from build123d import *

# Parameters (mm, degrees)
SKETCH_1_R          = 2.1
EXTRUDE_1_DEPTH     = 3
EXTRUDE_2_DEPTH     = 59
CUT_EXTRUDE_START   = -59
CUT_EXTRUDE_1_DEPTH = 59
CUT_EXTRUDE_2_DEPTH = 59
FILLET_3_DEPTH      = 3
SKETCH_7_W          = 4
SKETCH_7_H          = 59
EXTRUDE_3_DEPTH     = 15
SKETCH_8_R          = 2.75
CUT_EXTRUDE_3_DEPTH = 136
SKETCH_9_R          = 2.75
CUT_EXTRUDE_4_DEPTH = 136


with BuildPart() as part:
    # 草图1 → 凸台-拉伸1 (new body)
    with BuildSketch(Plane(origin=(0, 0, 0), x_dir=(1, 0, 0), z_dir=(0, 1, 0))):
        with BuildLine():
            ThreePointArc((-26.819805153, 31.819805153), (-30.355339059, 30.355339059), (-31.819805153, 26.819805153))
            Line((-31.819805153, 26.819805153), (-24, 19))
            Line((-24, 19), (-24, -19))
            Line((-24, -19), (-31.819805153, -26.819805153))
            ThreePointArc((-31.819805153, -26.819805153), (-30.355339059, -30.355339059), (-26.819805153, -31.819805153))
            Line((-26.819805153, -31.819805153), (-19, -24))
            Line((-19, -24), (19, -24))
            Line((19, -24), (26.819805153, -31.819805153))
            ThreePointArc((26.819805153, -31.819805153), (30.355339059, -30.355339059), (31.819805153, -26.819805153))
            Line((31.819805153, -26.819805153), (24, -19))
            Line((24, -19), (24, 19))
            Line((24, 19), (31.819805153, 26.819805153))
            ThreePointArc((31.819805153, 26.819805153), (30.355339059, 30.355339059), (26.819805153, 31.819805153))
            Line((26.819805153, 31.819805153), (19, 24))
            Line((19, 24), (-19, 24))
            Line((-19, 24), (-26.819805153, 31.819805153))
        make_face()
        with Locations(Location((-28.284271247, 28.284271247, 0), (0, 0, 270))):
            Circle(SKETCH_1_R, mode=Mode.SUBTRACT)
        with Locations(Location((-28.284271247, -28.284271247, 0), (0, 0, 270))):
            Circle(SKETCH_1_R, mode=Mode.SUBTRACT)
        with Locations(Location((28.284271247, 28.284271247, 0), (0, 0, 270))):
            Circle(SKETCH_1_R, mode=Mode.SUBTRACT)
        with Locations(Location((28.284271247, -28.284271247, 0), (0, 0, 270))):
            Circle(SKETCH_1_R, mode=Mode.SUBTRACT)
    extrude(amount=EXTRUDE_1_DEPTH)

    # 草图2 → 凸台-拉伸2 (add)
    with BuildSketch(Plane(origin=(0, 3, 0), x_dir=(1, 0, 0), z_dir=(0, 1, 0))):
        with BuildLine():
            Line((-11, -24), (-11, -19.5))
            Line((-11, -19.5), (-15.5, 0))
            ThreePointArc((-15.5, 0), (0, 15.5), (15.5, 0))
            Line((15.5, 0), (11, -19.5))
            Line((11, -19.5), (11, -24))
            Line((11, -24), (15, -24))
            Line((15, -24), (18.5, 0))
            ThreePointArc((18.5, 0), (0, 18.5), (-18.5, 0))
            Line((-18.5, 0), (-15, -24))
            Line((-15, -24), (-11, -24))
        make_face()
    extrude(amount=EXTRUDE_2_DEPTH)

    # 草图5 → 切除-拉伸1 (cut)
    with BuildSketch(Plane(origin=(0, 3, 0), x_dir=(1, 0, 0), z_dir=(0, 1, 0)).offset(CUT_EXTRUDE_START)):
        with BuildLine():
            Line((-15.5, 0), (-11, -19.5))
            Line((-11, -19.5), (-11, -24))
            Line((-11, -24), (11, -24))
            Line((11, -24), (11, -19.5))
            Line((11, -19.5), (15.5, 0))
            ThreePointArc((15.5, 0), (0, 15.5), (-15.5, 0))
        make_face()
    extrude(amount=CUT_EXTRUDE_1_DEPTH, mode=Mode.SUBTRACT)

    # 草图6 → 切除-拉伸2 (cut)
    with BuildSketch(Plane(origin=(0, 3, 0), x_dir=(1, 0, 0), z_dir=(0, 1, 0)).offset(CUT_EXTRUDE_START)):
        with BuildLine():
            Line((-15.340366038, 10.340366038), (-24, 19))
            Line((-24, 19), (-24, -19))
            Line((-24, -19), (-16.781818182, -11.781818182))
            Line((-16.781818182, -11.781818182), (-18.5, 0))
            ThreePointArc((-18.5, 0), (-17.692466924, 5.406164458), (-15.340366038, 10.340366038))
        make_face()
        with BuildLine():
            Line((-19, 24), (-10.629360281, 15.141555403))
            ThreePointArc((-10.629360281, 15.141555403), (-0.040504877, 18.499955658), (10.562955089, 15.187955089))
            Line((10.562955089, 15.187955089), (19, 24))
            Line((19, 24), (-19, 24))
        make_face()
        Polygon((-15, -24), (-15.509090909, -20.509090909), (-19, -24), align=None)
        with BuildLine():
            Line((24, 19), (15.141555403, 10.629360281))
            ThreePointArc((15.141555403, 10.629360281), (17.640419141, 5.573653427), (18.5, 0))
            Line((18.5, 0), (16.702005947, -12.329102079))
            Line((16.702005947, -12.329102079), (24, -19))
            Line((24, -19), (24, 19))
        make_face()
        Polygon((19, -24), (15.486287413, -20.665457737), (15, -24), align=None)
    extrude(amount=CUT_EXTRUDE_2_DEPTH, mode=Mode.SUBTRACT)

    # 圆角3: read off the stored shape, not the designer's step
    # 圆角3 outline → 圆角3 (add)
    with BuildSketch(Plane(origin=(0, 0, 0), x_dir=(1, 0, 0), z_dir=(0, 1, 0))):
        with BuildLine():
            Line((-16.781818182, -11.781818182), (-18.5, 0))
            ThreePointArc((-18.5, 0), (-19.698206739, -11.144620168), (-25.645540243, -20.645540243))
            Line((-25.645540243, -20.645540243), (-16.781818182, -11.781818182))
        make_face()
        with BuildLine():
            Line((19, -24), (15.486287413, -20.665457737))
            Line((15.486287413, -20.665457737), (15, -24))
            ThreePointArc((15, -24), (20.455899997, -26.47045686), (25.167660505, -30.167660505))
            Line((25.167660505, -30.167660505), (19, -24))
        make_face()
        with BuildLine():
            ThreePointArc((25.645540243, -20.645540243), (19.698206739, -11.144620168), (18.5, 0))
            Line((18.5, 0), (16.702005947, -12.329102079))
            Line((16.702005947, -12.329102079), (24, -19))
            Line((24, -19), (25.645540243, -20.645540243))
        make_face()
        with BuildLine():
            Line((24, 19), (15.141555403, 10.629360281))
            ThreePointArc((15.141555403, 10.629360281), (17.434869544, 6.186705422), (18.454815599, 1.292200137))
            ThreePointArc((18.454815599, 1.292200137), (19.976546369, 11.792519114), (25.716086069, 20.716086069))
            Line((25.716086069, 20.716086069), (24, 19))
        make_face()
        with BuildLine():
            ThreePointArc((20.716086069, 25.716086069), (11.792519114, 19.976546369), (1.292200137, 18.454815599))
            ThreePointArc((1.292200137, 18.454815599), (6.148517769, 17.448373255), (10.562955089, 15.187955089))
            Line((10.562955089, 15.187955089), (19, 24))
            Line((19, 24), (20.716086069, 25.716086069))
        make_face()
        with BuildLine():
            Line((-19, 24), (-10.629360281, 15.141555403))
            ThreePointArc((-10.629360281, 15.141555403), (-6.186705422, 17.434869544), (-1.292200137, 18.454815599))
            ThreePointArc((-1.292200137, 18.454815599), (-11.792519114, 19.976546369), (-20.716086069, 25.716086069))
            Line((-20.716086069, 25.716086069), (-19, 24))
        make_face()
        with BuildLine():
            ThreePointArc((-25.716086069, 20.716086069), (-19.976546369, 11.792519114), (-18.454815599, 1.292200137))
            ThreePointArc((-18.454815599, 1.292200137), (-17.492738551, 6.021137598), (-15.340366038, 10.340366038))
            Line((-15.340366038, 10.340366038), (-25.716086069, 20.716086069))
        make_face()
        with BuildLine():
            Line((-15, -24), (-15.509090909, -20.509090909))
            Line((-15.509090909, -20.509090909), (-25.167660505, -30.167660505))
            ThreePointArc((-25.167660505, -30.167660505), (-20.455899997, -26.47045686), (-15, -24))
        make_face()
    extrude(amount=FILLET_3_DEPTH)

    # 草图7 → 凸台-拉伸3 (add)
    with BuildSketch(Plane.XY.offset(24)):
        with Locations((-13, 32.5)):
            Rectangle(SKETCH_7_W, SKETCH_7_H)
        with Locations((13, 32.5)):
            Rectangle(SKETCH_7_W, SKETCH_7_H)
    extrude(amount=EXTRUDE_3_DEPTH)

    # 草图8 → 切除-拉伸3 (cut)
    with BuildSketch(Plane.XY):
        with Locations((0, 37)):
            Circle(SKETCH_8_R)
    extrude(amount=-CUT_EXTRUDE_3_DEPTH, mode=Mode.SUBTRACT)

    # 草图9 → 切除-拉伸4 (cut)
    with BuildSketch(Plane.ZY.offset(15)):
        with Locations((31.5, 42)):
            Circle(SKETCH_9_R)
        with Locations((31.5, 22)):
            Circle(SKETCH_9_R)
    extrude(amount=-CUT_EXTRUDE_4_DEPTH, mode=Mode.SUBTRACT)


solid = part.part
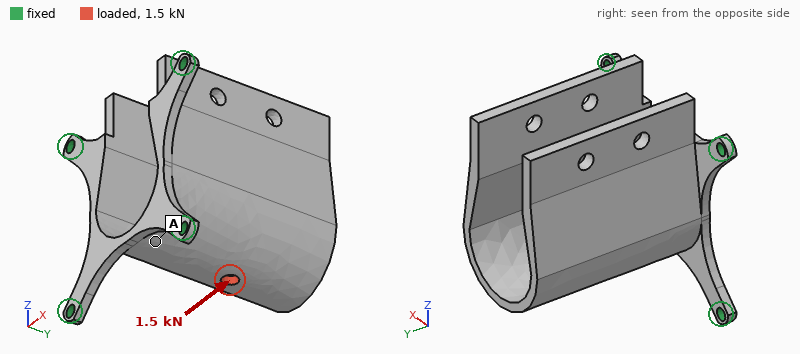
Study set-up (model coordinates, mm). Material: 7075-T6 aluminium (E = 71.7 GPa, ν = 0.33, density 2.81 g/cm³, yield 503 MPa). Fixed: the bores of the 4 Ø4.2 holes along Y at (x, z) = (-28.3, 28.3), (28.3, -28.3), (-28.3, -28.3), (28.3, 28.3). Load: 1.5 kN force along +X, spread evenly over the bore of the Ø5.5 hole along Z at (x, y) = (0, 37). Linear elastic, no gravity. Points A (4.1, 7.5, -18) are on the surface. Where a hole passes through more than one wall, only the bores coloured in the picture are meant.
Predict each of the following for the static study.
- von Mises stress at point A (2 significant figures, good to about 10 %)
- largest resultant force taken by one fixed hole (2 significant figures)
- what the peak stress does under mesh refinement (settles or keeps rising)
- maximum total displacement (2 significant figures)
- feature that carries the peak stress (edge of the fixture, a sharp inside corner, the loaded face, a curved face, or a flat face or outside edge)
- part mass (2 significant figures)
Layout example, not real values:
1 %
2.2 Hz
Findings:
41 MPa
930 N
keeps rising
1.1 mm
edge of the fixture
86 g
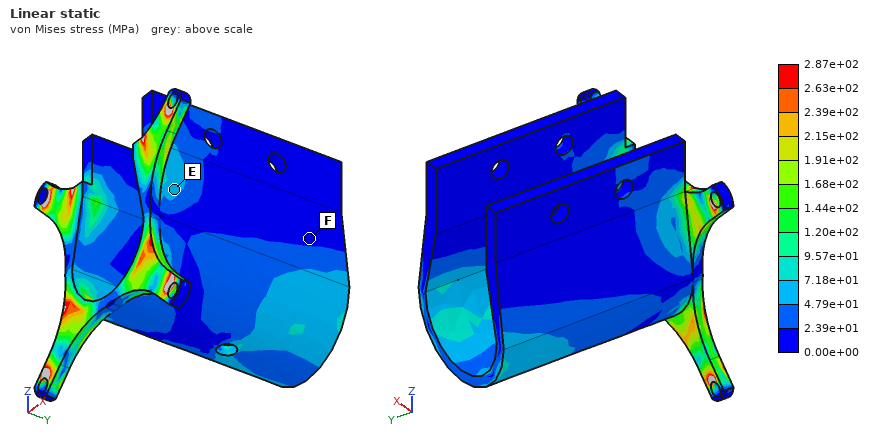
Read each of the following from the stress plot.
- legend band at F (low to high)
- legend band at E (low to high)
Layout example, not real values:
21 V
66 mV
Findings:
0.00e+00 to 2.39e+01 MPa
4.79e+01 to 7.18e+01 MPa
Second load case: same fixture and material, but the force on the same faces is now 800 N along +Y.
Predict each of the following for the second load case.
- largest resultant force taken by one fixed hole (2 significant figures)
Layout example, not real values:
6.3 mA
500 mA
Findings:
400 N
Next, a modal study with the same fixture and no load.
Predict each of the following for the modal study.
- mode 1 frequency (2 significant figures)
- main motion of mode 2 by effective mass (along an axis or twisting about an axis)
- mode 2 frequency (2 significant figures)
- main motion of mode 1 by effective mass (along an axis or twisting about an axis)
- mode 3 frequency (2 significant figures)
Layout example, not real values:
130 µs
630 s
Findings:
630 Hz
along Z
940 Hz
along X
1100 Hz
